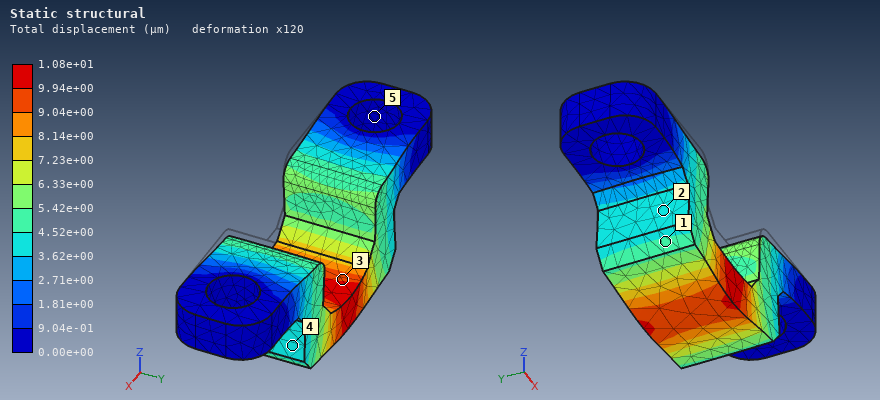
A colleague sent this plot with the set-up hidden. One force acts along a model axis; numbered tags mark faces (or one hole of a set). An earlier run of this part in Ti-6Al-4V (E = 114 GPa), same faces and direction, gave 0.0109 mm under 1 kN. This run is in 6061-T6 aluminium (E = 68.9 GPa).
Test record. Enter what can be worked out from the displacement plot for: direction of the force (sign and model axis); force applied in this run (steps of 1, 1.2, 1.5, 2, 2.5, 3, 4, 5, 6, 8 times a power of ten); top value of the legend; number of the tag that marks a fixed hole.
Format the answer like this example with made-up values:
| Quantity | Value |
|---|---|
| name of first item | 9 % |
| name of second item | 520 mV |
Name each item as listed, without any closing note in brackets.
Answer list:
| Quantity | Value |
|---|---|
| direction of the force | -Z |
| force applied in this run | 600 N |
| top value of the legend | 1.08e+01 µm |
| number of the tag that marks a fixed hole | 5 |
